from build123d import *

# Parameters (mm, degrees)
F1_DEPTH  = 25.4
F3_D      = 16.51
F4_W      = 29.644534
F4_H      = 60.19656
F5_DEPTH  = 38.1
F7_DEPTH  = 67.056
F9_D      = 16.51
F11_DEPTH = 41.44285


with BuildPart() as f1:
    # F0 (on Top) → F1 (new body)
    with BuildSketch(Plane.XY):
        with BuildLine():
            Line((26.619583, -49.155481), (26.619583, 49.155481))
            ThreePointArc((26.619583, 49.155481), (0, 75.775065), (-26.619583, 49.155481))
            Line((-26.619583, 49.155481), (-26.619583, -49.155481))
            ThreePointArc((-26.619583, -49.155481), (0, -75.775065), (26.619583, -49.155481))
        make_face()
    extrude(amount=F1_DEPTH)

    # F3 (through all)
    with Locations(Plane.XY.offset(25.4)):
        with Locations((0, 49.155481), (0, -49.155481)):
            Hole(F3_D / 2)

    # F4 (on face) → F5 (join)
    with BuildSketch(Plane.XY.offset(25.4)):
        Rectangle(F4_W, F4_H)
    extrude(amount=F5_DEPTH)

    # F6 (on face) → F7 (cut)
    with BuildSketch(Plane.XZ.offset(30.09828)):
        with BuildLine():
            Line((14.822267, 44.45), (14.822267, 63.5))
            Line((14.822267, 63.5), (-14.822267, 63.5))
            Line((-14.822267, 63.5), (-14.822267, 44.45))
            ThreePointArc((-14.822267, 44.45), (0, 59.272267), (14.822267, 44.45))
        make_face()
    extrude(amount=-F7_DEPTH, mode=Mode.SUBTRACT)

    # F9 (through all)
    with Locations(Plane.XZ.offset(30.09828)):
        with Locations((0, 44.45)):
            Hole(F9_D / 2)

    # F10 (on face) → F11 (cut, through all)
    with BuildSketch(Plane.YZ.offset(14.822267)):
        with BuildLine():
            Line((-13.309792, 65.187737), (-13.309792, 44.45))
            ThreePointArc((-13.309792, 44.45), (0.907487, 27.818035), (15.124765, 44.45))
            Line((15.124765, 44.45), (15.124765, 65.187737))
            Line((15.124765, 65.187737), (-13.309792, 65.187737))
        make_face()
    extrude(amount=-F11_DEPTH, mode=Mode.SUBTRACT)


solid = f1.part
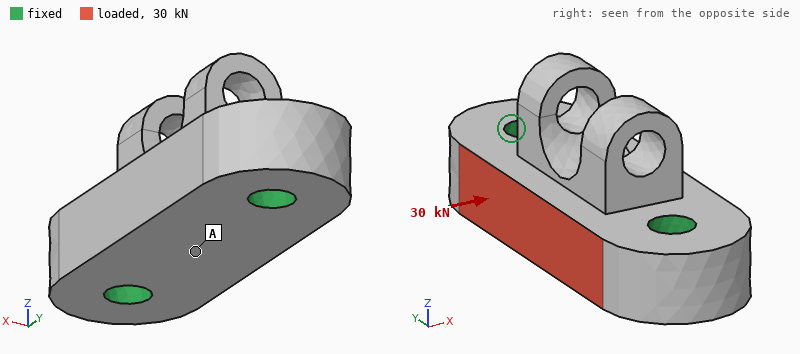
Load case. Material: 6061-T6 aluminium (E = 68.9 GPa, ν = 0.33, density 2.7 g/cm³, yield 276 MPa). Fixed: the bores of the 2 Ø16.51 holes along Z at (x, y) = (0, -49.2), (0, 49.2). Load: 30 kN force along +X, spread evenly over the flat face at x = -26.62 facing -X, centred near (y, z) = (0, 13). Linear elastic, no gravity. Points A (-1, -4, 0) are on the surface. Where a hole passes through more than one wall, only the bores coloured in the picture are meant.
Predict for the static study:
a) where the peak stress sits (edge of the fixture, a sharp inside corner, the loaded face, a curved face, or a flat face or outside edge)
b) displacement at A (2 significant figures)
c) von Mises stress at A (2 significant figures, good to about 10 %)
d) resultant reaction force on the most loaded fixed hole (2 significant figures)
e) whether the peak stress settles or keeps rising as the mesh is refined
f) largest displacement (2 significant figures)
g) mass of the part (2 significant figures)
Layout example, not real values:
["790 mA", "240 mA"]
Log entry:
["edge of the fixture", "17 µm", "6.8 MPa", "15 kN", "keeps rising", "20 µm", "550 g"]
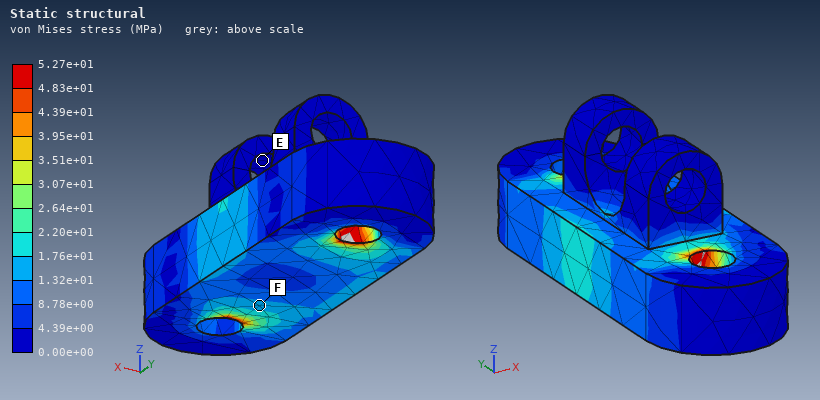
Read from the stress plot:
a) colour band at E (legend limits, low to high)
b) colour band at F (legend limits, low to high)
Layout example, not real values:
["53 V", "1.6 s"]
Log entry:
["0.00e+00 to 4.39e+00 MPa", "1.32e+01 to 1.76e+01 MPa"]
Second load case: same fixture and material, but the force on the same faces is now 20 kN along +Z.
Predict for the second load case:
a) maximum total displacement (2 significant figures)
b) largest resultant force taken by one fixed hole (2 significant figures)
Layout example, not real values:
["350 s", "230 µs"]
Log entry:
["53 µm", "10 kN"]
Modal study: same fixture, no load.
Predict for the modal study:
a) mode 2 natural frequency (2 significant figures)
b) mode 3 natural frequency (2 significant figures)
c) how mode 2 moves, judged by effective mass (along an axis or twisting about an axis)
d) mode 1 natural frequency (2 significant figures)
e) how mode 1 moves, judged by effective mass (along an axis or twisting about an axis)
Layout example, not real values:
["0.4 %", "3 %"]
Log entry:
["9100 Hz", "11 kHz", "along Z", "8200 Hz", "along X"]
